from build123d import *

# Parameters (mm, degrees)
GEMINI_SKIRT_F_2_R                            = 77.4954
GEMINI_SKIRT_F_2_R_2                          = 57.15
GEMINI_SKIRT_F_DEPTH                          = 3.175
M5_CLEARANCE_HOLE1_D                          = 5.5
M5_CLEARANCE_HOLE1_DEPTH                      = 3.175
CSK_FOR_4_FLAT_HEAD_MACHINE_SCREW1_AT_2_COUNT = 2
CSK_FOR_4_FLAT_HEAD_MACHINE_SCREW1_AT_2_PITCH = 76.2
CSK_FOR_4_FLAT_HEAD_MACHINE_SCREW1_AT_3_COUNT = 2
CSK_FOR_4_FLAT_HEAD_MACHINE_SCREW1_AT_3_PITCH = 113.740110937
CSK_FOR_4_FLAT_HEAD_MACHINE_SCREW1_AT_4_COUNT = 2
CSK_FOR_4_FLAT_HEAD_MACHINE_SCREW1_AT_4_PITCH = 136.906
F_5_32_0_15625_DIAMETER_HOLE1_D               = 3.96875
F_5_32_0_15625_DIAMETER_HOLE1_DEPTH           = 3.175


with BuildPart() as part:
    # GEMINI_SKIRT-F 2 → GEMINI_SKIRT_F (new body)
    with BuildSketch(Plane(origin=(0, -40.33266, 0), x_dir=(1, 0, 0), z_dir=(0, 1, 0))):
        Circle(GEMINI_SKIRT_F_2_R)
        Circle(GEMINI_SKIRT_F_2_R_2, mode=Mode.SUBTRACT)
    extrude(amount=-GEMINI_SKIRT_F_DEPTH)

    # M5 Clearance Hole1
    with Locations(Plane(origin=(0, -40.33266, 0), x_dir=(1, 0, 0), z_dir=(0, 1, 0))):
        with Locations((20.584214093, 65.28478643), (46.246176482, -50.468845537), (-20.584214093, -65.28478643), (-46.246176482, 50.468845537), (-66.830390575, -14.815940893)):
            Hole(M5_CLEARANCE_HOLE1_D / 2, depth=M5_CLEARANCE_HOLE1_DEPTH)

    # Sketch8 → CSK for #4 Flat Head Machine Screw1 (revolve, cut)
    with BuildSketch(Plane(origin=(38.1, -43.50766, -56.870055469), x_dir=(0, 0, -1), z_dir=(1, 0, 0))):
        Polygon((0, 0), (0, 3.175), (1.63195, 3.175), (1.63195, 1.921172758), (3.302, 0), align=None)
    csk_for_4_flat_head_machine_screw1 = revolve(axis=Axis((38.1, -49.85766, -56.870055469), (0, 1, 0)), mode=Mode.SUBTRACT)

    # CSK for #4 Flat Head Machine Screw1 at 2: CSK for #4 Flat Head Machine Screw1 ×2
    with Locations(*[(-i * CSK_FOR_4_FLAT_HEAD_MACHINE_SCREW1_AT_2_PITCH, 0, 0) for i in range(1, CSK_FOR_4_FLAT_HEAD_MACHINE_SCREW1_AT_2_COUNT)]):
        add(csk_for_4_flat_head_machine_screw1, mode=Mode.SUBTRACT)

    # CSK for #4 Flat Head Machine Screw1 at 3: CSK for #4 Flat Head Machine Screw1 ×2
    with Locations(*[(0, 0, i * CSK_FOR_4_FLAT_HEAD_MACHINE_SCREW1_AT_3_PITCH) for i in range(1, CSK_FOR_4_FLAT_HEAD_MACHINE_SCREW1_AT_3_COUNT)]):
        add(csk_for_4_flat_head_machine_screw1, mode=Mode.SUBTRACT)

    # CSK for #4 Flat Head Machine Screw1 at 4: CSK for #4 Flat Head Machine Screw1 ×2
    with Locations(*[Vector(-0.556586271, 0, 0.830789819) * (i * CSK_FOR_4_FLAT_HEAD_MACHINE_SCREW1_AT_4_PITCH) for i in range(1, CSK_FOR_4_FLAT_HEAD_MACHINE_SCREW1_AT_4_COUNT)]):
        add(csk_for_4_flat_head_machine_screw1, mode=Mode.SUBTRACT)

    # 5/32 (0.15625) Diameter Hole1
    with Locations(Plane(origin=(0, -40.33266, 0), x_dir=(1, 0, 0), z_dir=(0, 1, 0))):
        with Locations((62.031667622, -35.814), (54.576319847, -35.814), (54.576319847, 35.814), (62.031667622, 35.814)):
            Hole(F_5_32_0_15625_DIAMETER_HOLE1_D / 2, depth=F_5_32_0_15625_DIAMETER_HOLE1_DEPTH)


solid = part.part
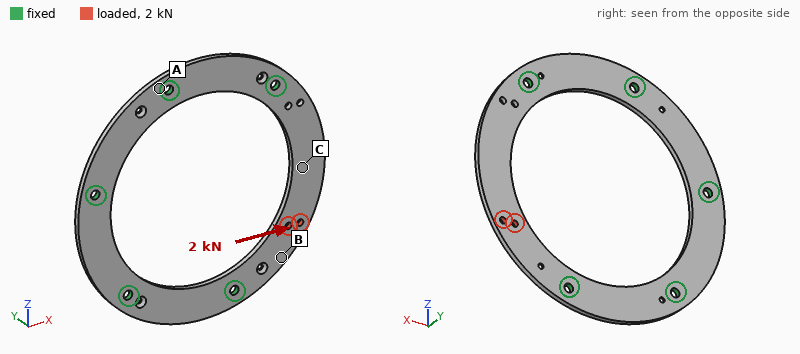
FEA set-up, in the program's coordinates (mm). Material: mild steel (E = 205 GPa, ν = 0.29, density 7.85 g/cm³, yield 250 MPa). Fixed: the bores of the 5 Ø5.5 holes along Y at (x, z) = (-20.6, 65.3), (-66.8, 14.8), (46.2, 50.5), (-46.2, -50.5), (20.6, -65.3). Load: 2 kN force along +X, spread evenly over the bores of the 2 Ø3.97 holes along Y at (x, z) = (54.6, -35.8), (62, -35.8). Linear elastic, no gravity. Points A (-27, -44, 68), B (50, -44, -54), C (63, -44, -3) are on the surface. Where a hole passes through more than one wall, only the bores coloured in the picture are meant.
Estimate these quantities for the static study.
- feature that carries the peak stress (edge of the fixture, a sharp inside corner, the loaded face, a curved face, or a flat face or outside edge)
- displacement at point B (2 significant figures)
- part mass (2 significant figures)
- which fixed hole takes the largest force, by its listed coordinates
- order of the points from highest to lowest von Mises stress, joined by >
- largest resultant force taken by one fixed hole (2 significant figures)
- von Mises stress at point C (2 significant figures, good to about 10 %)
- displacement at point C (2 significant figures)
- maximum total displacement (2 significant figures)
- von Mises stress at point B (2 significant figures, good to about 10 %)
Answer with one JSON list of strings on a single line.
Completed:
["the loaded face", "11 µm", "210 g", "(20.6, -65.3)", "B > C > A", "1.9 kN", "19 MPa", "9.0 µm", "21 µm", "30 MPa"]
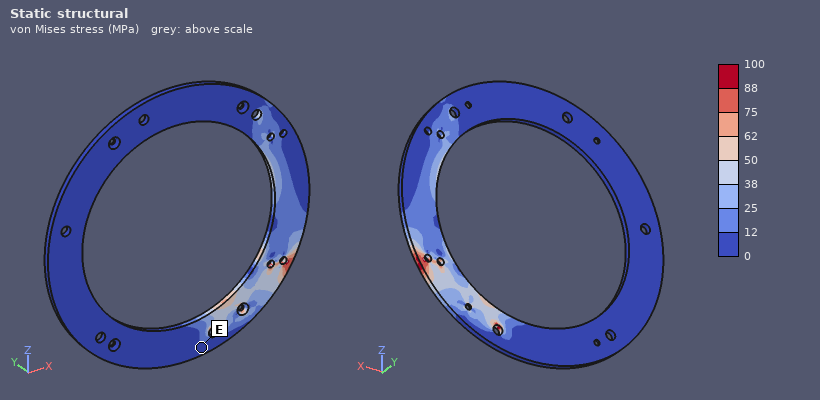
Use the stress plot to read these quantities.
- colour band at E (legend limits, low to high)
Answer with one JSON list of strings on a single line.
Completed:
["0 to 12 MPa"]
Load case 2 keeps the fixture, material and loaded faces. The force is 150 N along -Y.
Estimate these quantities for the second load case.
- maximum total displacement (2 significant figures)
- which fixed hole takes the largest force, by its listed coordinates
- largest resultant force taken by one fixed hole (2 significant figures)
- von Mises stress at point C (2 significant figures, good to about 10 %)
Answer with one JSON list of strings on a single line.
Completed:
["0.24 mm", "(20.6, -65.3)", "110 N", "19 MPa"]
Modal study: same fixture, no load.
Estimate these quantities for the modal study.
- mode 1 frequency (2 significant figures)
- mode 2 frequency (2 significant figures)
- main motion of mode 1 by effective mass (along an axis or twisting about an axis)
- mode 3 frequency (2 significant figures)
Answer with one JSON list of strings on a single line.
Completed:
["750 Hz", "2200 Hz", "along Y", "3300 Hz"]
